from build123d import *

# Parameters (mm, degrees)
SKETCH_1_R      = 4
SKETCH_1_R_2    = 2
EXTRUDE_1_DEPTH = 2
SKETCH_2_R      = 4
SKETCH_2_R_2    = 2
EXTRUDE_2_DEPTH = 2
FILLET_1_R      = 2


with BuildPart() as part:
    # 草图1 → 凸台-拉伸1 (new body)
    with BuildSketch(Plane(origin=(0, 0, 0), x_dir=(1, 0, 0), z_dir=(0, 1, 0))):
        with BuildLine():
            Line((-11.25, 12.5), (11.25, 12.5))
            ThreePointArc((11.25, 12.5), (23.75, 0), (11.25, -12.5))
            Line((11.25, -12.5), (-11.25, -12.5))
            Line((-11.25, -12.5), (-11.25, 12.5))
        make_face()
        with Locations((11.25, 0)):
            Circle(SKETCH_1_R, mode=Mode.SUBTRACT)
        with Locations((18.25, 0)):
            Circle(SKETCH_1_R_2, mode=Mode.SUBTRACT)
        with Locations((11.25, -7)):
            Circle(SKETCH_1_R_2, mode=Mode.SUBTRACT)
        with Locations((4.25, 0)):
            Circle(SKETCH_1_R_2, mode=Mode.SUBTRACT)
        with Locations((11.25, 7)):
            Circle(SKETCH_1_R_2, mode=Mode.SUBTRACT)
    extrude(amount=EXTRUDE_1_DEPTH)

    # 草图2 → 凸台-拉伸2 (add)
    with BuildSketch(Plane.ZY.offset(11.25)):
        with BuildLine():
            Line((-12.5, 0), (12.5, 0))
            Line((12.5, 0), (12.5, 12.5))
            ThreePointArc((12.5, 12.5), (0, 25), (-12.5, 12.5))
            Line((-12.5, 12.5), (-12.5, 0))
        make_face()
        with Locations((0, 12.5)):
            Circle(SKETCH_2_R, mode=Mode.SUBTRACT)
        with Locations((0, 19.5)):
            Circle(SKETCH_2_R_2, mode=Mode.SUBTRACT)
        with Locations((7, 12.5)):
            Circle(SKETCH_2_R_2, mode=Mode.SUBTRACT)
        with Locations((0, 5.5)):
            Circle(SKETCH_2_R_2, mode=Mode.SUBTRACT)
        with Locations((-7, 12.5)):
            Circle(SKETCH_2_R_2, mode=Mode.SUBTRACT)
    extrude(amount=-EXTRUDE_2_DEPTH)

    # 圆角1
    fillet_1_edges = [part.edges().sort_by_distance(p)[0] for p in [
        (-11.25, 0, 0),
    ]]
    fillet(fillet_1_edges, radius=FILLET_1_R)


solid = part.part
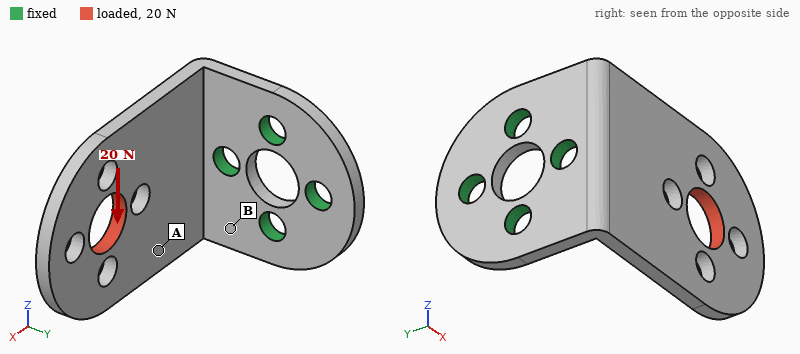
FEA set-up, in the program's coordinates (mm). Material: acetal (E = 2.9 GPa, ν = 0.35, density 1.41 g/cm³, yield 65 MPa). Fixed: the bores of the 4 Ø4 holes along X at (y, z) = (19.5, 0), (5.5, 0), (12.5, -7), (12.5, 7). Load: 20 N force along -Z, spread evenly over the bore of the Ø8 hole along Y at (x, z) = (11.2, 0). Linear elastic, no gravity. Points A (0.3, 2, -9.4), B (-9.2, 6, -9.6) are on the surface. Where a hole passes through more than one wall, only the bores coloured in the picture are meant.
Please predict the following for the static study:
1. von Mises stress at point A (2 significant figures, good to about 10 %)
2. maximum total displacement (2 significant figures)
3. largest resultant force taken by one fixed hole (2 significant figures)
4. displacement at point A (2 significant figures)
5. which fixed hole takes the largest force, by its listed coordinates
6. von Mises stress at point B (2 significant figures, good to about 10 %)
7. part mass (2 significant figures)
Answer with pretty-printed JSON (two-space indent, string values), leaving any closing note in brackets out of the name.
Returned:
{
  "von Mises stress at point A": "2.7 MPa",
  "maximum total displacement": "0.54 mm",
  "largest resultant force taken by one fixed hole": "17 N",
  "displacement at point A": "0.23 mm",
  "which fixed hole takes the largest force, by its listed coordinates": "(5.5, 0)",
  "von Mises stress at point B": "6.6 MPa",
  "part mass": "3.1 g"
}
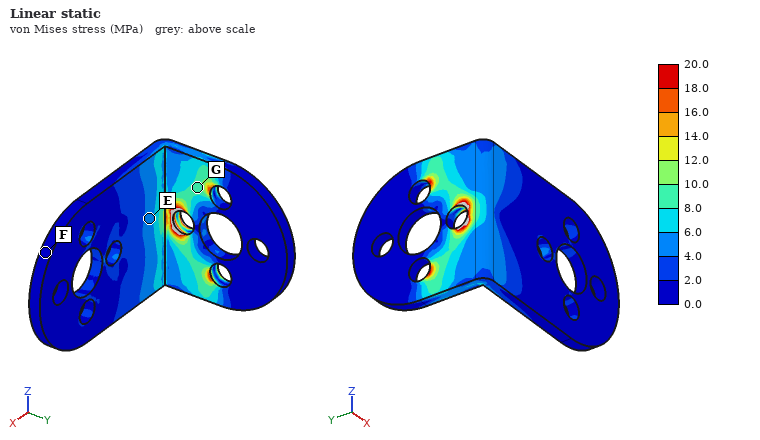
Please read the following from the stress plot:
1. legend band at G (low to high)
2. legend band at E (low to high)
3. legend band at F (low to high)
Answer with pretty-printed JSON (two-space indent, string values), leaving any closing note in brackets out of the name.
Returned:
{
  "legend band at G": "8.0 to 10.0 MPa",
  "legend band at E": "4.0 to 6.0 MPa",
  "legend band at F": "0.0 to 2.0 MPa"
}
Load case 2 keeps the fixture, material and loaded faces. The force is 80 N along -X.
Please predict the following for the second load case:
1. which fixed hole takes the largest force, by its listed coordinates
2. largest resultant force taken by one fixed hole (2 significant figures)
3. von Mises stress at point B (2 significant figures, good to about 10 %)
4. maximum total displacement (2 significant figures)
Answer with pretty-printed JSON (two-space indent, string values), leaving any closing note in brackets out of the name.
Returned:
{
  "which fixed hole takes the largest force, by its listed coordinates": "(5.5, 0)",
  "largest resultant force taken by one fixed hole": "85 N",
  "von Mises stress at point B": "4.0 MPa",
  "maximum total displacement": "0.49 mm"
}
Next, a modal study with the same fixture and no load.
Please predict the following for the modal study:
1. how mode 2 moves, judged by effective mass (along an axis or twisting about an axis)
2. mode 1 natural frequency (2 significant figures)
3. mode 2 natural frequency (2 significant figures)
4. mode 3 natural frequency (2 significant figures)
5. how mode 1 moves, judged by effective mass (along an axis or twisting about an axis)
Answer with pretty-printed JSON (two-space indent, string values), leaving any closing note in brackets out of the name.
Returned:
{
  "how mode 2 moves, judged by effective mass": "along Z",
  "mode 1 natural frequency": "430 Hz",
  "mode 2 natural frequency": "950 Hz",
  "mode 3 natural frequency": "1400 Hz",
  "how mode 1 moves, judged by effective mass": "along Y"
}
